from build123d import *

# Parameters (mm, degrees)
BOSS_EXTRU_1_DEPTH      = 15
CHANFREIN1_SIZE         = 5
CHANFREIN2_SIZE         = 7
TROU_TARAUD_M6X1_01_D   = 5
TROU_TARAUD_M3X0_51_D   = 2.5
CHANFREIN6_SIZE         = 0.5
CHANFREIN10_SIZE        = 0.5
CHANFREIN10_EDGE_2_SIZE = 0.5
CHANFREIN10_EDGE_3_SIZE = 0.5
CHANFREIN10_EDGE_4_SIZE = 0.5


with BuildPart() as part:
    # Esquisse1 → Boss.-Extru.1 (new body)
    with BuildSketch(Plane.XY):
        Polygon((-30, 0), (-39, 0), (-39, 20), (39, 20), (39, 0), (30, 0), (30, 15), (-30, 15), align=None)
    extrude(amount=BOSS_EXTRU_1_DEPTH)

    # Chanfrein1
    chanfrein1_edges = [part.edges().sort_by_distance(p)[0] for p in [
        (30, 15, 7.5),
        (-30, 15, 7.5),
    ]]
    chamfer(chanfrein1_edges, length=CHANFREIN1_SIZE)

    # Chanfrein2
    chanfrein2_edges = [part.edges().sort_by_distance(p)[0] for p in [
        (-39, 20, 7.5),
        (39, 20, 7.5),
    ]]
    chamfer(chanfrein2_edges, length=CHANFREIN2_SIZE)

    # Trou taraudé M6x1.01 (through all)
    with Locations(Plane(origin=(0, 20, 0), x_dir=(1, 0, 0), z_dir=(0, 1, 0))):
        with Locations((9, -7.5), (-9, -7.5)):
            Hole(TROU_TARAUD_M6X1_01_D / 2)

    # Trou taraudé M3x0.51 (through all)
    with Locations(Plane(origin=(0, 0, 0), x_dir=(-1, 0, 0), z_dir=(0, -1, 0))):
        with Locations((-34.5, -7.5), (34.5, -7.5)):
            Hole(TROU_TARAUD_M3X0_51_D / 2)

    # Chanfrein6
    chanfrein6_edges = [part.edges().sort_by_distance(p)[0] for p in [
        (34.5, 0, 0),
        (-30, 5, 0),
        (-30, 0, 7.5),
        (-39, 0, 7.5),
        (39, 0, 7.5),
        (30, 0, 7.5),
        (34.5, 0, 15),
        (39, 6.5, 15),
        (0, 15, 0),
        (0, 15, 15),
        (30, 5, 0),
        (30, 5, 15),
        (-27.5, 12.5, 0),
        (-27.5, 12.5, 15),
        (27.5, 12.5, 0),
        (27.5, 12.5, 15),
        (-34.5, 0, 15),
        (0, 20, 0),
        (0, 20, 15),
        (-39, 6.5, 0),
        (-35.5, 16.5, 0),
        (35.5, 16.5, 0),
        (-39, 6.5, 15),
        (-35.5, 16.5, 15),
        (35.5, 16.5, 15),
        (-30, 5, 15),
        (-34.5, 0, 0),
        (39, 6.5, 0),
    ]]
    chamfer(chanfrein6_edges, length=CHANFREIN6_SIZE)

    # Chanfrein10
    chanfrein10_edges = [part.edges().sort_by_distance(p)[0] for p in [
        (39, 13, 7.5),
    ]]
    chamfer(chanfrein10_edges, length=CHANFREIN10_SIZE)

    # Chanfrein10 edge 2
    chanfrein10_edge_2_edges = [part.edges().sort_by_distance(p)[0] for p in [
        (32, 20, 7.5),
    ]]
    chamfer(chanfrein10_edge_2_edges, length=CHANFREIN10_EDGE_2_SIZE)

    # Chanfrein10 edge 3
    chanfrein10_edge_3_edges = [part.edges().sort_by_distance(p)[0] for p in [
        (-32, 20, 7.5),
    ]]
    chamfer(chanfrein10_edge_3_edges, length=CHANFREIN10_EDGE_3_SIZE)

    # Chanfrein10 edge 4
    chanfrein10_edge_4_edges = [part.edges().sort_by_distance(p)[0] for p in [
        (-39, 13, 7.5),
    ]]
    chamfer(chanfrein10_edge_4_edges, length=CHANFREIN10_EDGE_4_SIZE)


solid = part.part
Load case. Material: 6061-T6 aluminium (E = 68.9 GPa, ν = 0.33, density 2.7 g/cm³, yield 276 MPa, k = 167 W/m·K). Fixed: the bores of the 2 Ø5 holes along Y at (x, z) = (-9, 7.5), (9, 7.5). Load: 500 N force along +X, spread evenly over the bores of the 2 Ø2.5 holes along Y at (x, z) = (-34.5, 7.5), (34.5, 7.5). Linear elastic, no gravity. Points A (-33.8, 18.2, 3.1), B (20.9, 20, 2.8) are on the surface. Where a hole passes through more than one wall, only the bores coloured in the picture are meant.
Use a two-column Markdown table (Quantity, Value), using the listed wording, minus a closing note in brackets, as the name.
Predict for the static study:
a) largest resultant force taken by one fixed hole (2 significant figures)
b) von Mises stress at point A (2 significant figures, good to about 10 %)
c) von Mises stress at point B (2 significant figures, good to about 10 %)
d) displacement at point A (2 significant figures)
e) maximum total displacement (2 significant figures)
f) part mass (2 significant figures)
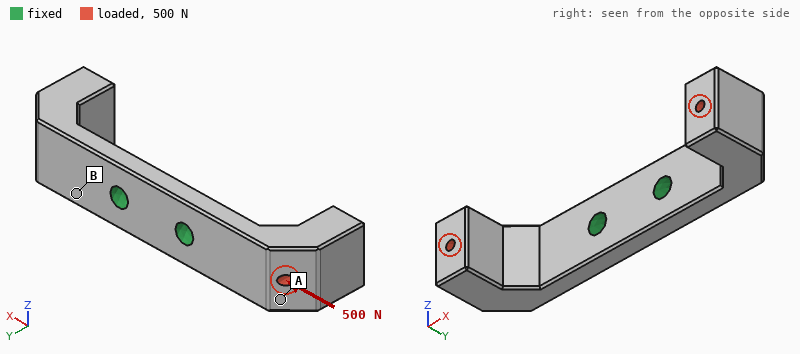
| Quantity | Value |
|---|---|
| largest resultant force taken by one fixed hole | 250 N |
| von Mises stress at point A | 6.5 MPa |
| von Mises stress at point B | 32 MPa |
| displacement at point A | 53 µm |
| maximum total displacement | 97 µm |
| part mass | 25 g |
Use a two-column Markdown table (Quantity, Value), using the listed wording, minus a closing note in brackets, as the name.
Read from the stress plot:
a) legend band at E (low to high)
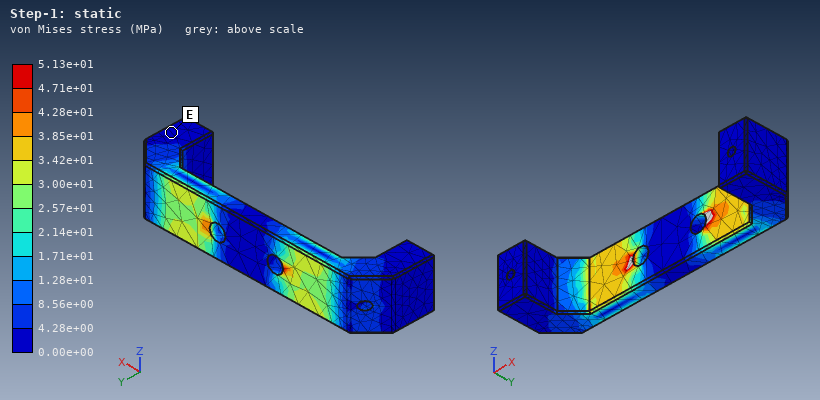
| Quantity | Value |
|---|---|
| legend band at E | 0.00e+00 to 4.28e+00 MPa |
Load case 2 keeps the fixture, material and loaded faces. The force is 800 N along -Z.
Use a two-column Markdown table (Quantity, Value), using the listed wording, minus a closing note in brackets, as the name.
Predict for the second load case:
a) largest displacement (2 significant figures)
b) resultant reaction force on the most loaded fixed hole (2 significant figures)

| Quantity | Value |
|---|---|
| largest displacement | 0.12 mm |
| resultant reaction force on the most loaded fixed hole | 400 N |
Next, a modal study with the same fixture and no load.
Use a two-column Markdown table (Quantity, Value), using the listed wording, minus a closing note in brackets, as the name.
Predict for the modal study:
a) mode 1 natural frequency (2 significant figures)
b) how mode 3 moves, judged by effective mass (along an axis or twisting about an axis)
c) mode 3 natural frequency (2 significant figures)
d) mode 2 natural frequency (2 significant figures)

| Quantity | Value |
|---|---|
| mode 1 natural frequency | 2500 Hz |
| how mode 3 moves, judged by effective mass | twisting about Y |
| mode 3 natural frequency | 4300 Hz |
| mode 2 natural frequency | 2500 Hz |
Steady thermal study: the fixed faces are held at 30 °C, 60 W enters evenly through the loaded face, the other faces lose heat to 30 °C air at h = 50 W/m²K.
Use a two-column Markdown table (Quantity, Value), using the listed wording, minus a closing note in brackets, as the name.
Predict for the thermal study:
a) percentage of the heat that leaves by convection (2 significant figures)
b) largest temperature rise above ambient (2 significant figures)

| Quantity | Value |
|---|---|
| percentage of the heat that leaves by convection | 11 % |
| largest temperature rise above ambient | 55 K |
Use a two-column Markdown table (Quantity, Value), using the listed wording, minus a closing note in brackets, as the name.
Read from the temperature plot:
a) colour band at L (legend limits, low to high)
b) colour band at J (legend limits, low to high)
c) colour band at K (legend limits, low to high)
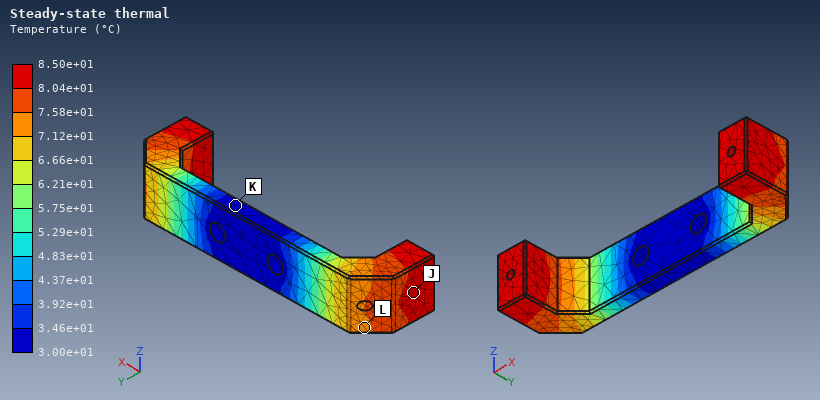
| Quantity | Value |
|---|---|
| colour band at L | 7.12e+01 to 7.58e+01 °C |
| colour band at J | 8.04e+01 to 8.50e+01 °C |
| colour band at K | 3.00e+01 to 3.46e+01 °C |
